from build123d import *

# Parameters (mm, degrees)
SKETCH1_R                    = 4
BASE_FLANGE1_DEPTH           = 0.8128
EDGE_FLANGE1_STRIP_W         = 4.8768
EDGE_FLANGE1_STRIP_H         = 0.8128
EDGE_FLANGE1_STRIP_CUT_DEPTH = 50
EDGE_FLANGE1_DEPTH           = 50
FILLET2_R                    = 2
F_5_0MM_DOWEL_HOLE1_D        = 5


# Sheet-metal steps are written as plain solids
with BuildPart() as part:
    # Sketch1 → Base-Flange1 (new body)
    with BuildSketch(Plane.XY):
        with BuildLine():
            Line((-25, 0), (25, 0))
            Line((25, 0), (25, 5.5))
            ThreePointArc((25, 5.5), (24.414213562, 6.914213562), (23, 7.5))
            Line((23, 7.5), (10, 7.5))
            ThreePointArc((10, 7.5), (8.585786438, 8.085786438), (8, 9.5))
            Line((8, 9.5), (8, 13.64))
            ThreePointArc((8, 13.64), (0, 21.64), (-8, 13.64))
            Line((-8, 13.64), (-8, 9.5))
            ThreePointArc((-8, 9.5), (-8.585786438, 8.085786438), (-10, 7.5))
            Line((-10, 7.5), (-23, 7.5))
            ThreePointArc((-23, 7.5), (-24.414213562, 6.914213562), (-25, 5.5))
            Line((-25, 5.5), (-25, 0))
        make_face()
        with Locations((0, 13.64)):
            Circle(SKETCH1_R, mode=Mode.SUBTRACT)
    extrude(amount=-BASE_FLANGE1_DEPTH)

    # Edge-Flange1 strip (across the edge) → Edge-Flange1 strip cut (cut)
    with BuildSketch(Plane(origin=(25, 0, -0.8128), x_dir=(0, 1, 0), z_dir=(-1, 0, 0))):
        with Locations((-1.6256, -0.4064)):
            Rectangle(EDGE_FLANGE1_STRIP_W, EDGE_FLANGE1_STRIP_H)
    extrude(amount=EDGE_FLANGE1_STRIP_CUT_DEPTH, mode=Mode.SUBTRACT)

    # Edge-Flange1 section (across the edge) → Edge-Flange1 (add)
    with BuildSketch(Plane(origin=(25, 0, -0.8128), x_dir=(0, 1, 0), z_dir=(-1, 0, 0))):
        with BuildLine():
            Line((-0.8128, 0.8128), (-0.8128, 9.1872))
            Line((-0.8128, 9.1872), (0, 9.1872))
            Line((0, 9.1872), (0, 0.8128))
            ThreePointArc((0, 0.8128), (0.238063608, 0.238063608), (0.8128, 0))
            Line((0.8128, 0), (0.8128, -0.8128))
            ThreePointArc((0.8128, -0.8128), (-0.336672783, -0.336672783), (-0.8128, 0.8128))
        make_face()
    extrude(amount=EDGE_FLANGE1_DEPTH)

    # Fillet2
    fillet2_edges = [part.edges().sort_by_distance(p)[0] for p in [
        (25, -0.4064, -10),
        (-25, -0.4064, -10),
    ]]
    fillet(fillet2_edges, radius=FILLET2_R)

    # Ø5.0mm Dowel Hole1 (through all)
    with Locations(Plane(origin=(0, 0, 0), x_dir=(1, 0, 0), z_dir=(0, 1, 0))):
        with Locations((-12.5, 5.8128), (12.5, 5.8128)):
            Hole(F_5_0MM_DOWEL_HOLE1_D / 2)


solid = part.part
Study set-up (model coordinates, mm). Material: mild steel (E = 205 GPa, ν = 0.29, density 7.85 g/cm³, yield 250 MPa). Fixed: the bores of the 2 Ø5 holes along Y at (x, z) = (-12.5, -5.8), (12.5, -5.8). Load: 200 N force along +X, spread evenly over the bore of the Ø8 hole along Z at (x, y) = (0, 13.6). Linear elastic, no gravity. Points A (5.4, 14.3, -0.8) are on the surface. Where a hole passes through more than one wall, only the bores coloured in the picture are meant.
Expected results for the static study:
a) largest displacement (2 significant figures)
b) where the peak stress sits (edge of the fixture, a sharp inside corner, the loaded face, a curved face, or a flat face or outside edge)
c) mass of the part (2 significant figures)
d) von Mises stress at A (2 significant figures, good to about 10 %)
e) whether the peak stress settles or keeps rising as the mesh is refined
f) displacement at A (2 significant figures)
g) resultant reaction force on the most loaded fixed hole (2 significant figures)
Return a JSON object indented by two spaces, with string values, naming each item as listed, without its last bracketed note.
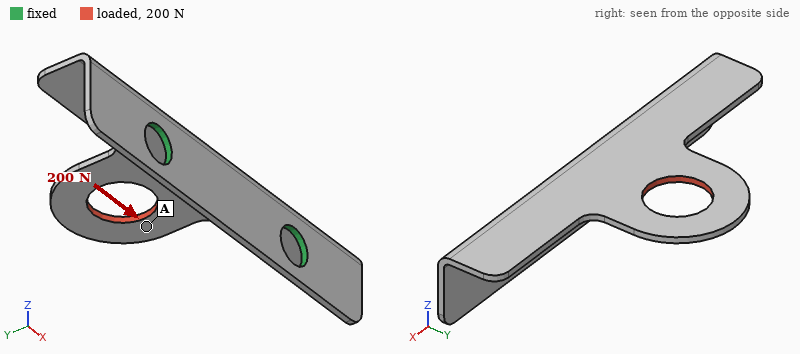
{
  "largest displacement": "37 µm",
  "where the peak stress sits": "edge of the fixture",
  "mass of the part": "6.1 g",
  "von Mises stress at A": "43 MPa",
  "whether the peak stress settles or keeps rising as the mesh is refined": "keeps rising",
  "displacement at A": "26 µm",
  "resultant reaction force on the most loaded fixed hole": "150 N"
}
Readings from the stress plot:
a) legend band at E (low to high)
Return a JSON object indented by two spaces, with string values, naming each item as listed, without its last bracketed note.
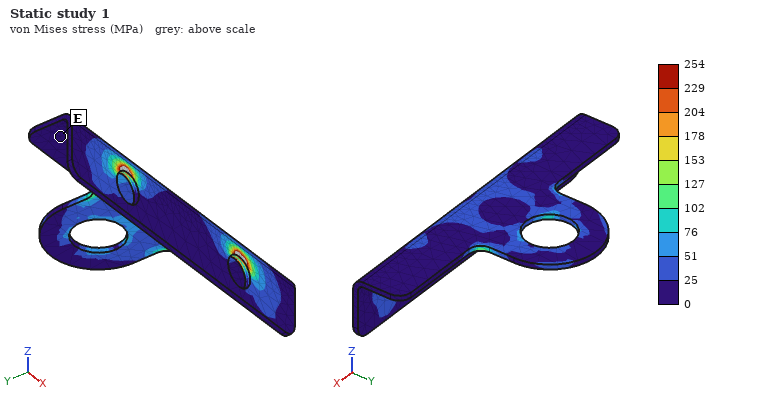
{
  "legend band at E": "0 to 25 MPa"
}
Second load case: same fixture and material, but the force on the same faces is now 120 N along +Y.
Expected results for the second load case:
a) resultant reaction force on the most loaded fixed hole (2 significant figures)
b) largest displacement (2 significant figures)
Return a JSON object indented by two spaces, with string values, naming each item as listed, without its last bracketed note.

{
  "resultant reaction force on the most loaded fixed hole": "68 N",
  "largest displacement": "53 µm"
}
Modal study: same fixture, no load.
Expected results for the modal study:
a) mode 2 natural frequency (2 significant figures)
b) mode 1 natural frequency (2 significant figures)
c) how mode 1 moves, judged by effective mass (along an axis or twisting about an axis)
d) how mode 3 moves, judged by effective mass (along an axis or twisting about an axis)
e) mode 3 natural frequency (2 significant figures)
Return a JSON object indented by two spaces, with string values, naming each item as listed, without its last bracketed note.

{
  "mode 2 natural frequency": "5100 Hz",
  "mode 1 natural frequency": "1800 Hz",
  "how mode 1 moves, judged by effective mass": "along Z",
  "how mode 3 moves, judged by effective mass": "along Z",
  "mode 3 natural frequency": "6300 Hz"
}
